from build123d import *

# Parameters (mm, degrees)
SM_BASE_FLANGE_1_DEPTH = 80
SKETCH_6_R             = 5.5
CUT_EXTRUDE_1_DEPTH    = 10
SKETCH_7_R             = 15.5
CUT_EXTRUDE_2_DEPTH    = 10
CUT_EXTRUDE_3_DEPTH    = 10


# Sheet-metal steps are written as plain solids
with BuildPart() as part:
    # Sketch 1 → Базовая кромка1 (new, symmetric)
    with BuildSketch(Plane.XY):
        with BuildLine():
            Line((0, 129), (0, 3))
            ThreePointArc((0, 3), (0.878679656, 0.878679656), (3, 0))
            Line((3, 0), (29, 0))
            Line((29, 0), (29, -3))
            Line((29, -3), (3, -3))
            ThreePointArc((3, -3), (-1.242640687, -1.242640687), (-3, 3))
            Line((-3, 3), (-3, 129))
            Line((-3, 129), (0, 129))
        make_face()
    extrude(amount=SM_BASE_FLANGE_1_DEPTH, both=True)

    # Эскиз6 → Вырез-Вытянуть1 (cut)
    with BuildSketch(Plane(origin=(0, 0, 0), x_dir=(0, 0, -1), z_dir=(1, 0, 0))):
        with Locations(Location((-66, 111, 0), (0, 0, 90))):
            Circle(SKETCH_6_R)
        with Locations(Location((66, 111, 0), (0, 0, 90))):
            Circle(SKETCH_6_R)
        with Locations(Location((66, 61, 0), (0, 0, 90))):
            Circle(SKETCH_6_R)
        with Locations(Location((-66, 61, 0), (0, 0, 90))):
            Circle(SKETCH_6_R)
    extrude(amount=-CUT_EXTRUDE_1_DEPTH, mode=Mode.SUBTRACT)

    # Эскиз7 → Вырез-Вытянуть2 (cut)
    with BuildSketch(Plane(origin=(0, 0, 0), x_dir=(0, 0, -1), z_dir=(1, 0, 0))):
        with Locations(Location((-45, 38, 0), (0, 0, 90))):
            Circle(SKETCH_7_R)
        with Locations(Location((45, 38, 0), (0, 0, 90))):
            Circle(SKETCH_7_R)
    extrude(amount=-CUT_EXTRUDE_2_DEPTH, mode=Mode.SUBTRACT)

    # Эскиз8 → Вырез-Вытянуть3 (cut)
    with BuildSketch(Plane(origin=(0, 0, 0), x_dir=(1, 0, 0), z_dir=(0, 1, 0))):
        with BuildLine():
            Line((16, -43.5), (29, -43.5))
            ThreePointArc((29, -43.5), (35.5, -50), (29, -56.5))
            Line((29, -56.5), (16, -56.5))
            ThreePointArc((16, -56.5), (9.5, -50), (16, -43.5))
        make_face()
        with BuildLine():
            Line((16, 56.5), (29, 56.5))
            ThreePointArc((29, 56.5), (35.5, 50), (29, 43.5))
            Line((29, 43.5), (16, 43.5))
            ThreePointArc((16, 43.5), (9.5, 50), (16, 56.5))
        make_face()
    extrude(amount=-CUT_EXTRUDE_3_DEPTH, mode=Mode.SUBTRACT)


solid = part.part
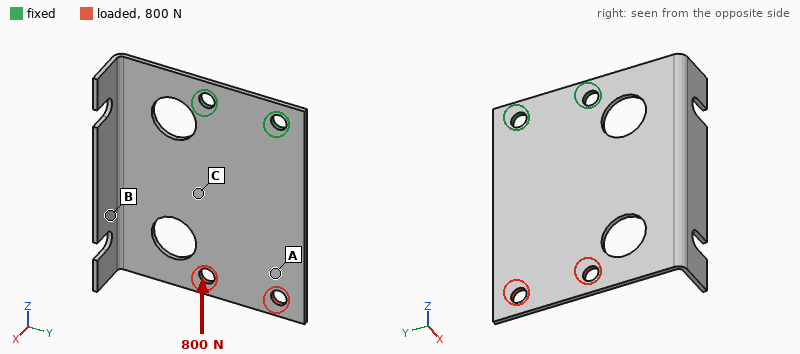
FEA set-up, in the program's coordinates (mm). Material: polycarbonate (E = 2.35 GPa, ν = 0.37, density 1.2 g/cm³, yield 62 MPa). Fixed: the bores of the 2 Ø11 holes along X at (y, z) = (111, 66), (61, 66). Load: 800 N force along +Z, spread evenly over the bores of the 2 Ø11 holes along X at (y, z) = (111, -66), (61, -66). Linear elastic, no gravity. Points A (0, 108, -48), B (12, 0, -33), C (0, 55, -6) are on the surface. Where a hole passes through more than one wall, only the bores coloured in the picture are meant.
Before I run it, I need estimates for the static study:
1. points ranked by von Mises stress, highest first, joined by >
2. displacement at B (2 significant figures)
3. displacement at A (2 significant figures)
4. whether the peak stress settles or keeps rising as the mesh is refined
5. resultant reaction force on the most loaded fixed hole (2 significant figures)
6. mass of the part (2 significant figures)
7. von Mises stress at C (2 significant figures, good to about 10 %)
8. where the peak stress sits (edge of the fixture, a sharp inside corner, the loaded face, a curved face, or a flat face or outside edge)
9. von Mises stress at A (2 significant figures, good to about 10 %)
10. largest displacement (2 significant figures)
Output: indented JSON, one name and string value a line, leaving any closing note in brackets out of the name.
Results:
{
  "points ranked by von Mises stress, highest first, joined by >": "A > C > B",
  "displacement at B": "0.12 mm",
  "displacement at A": "0.17 mm",
  "whether the peak stress settles or keeps rising as the mesh is refined": "keeps rising",
  "resultant reaction force on the most loaded fixed hole": "410 N",
  "mass of the part": "83 g",
  "von Mises stress at C": "2.3 MPa",
  "where the peak stress sits": "a sharp inside corner",
  "von Mises stress at A": "3.6 MPa",
  "largest displacement": "0.24 mm"
}
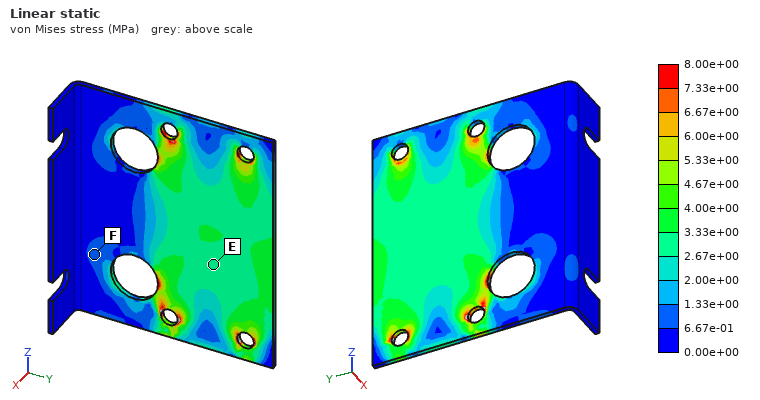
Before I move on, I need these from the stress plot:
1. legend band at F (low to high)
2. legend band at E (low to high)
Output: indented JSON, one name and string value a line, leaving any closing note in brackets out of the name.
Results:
{
  "legend band at F": "6.67e-01 to 1.33e+00 MPa",
  "legend band at E": "2.67e+00 to 3.33e+00 MPa"
}
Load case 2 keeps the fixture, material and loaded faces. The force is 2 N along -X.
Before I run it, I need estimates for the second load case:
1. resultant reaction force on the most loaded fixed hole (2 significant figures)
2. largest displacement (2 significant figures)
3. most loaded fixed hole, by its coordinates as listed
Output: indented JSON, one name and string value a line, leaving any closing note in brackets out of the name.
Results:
{
  "resultant reaction force on the most loaded fixed hole": "1.4 N",
  "largest displacement": "2.5 mm",
  "most loaded fixed hole, by its coordinates as listed": "(61, 66)"
}
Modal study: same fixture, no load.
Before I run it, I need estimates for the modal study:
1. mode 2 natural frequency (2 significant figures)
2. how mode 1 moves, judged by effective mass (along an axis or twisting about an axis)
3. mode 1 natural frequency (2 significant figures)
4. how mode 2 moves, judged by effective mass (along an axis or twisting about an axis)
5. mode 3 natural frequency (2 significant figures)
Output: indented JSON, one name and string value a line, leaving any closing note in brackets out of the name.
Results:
{
  "mode 2 natural frequency": "59 Hz",
  "how mode 1 moves, judged by effective mass": "along X",
  "mode 1 natural frequency": "29 Hz",
  "how mode 2 moves, judged by effective mass": "twisting about Z",
  "mode 3 natural frequency": "120 Hz"
}
